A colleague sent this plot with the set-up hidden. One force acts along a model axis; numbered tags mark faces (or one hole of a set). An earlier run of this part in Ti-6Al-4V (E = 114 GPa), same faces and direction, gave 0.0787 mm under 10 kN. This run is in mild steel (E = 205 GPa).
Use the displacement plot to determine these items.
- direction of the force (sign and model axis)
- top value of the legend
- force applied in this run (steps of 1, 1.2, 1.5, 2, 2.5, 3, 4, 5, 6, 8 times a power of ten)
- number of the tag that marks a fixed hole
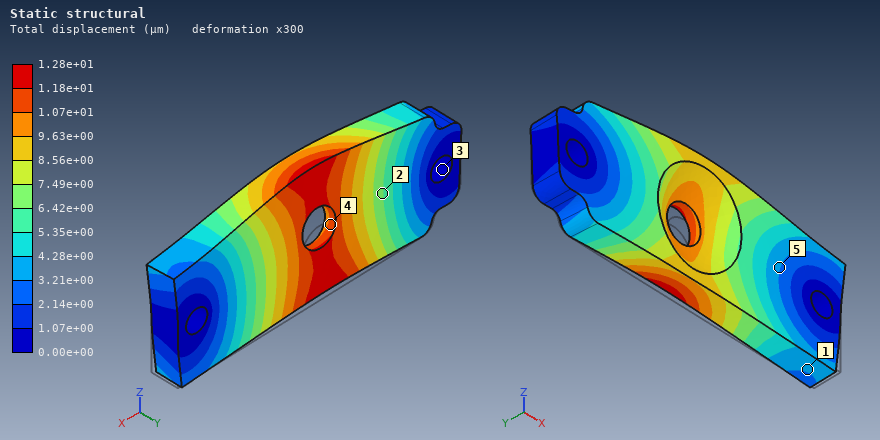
+Z
1.28e+01 µm
3 kN
3
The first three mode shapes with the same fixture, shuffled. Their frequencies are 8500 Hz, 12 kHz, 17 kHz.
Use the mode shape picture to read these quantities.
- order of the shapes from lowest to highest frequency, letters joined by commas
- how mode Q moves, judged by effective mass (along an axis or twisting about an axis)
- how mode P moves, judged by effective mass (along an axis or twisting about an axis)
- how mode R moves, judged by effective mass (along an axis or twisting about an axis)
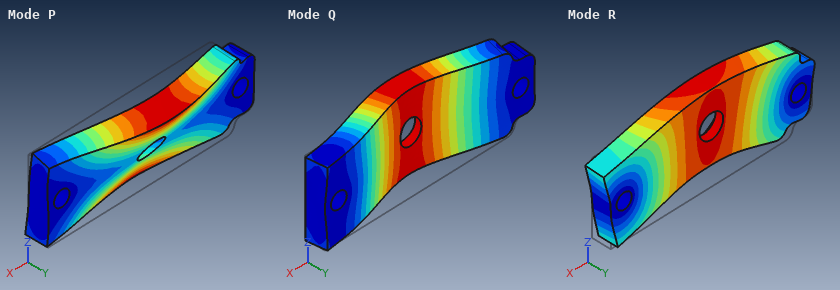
Q, P, R
along Y
twisting about X
along Z
